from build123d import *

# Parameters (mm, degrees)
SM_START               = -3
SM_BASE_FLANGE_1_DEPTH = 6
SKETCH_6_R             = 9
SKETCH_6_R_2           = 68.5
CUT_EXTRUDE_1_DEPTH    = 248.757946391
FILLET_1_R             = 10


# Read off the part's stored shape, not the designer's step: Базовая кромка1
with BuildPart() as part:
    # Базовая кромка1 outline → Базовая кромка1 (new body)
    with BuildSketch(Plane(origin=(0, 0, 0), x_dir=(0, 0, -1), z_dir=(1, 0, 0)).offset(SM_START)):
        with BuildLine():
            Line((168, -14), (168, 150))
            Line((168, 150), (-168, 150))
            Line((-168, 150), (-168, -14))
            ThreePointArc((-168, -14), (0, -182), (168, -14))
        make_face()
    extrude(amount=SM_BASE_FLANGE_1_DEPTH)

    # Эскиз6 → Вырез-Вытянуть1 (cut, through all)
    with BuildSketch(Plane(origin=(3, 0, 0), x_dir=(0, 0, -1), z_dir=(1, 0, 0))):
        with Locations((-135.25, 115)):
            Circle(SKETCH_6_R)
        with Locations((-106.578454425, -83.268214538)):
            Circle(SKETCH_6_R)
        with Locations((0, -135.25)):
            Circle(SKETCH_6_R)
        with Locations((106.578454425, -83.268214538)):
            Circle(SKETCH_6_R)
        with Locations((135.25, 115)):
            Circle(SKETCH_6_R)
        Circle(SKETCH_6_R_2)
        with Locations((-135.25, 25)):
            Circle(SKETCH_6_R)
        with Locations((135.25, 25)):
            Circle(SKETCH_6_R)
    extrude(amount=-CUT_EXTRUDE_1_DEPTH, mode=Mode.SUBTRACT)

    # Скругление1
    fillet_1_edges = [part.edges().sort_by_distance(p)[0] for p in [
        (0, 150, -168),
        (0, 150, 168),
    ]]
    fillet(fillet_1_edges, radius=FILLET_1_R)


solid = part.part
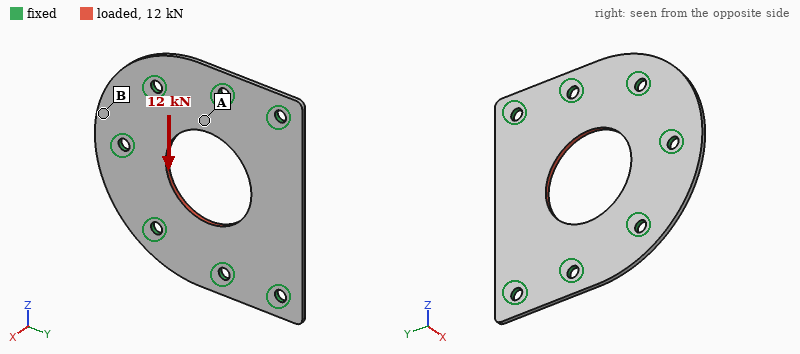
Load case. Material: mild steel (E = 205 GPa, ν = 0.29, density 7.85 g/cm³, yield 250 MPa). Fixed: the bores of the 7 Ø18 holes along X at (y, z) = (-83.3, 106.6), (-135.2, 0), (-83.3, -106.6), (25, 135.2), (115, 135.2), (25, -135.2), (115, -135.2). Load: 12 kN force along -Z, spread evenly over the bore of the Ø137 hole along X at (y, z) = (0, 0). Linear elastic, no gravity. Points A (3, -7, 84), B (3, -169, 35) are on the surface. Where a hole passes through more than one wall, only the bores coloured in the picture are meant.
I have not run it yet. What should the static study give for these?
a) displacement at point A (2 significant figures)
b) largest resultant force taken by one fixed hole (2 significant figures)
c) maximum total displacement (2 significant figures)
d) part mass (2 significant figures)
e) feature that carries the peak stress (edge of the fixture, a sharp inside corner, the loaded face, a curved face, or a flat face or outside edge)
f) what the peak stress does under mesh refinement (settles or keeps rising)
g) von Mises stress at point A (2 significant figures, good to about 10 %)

1.7 µm
2.3 kN
2.8 µm
3.9 kg
edge of the fixture
keeps rising
4.3 MPa
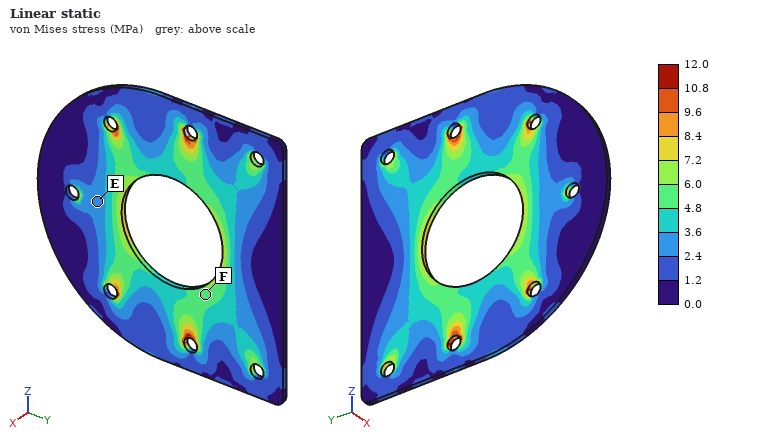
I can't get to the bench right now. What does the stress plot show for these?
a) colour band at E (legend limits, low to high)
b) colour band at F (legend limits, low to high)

2.4 to 3.6 MPa
4.8 to 6.0 MPa
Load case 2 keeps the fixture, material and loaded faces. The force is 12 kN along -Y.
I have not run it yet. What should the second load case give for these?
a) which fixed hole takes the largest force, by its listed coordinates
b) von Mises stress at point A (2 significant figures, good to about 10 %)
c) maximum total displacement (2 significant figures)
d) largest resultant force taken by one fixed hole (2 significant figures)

(-135.2, 0)
6.9 MPa
6.2 µm
2.5 kN
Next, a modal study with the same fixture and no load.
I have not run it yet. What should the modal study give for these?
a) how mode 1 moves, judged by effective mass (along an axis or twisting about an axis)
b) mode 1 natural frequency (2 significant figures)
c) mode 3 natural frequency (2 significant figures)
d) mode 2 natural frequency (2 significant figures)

along X
510 Hz
1200 Hz
1100 Hz
